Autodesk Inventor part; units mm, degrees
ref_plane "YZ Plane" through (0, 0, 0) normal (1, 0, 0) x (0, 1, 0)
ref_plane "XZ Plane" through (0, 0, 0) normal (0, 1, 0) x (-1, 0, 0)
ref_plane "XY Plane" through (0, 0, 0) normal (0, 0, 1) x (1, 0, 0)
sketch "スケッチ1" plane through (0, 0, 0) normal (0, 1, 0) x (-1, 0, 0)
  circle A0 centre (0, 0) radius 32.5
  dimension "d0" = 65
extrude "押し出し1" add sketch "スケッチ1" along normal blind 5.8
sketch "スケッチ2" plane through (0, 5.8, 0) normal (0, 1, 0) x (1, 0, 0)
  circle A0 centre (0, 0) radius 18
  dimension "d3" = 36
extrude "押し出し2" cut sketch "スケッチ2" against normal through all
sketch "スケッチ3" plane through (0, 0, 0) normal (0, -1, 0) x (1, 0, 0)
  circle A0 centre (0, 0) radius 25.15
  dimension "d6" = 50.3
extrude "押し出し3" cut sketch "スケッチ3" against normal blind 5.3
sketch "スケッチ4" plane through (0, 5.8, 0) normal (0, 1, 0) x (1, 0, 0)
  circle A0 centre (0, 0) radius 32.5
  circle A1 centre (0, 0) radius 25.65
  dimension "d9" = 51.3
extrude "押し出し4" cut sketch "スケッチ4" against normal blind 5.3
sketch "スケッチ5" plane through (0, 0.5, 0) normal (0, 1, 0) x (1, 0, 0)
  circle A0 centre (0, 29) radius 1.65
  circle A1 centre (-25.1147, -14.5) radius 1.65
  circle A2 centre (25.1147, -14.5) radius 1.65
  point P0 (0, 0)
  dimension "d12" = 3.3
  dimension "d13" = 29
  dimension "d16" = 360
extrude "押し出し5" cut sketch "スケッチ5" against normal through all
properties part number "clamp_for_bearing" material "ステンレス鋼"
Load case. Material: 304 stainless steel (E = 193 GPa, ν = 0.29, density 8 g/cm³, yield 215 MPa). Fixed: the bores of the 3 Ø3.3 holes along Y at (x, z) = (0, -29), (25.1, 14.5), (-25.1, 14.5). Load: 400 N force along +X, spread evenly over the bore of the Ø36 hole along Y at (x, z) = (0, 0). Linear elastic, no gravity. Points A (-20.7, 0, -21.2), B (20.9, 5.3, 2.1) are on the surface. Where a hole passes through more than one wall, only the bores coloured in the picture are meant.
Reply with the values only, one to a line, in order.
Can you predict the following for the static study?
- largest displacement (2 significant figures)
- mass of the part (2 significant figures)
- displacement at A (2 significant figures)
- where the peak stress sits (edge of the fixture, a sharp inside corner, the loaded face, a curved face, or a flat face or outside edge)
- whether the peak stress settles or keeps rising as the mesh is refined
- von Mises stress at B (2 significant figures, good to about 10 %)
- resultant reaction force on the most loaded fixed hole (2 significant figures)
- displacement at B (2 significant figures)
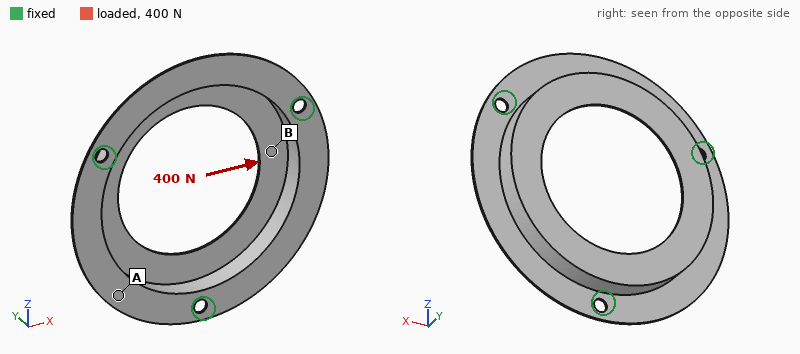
36 µm
12 g
29 µm
edge of the fixture
keeps rising
25 MPa
140 N
11 µm
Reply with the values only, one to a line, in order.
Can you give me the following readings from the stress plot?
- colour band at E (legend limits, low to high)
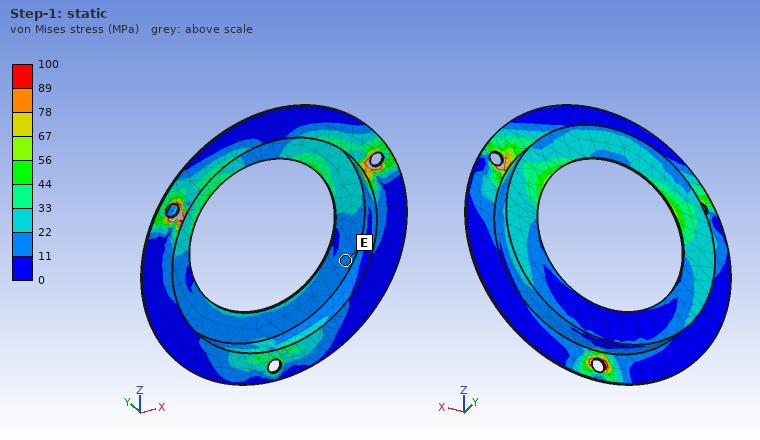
11 to 22 MPa
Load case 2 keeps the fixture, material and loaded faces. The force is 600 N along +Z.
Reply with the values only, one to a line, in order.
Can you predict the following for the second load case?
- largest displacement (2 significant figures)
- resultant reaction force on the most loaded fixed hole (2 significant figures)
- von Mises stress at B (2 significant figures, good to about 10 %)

62 µm
210 N
38 MPa
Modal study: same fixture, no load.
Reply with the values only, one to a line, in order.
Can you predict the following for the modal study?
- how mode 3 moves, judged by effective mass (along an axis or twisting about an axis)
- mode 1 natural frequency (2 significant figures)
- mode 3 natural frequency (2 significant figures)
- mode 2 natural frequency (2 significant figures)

along Y
3400 Hz
4600 Hz
3400 Hz
